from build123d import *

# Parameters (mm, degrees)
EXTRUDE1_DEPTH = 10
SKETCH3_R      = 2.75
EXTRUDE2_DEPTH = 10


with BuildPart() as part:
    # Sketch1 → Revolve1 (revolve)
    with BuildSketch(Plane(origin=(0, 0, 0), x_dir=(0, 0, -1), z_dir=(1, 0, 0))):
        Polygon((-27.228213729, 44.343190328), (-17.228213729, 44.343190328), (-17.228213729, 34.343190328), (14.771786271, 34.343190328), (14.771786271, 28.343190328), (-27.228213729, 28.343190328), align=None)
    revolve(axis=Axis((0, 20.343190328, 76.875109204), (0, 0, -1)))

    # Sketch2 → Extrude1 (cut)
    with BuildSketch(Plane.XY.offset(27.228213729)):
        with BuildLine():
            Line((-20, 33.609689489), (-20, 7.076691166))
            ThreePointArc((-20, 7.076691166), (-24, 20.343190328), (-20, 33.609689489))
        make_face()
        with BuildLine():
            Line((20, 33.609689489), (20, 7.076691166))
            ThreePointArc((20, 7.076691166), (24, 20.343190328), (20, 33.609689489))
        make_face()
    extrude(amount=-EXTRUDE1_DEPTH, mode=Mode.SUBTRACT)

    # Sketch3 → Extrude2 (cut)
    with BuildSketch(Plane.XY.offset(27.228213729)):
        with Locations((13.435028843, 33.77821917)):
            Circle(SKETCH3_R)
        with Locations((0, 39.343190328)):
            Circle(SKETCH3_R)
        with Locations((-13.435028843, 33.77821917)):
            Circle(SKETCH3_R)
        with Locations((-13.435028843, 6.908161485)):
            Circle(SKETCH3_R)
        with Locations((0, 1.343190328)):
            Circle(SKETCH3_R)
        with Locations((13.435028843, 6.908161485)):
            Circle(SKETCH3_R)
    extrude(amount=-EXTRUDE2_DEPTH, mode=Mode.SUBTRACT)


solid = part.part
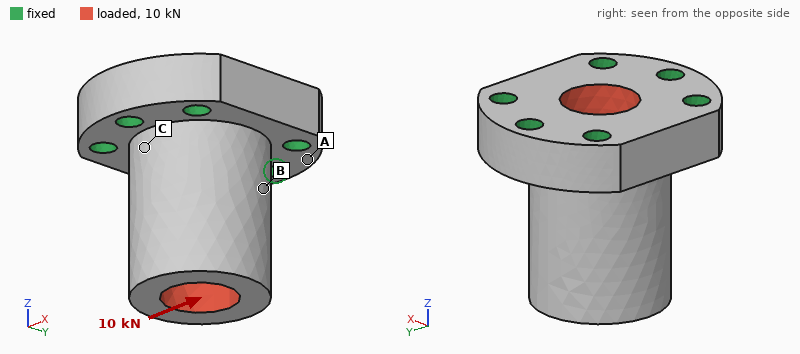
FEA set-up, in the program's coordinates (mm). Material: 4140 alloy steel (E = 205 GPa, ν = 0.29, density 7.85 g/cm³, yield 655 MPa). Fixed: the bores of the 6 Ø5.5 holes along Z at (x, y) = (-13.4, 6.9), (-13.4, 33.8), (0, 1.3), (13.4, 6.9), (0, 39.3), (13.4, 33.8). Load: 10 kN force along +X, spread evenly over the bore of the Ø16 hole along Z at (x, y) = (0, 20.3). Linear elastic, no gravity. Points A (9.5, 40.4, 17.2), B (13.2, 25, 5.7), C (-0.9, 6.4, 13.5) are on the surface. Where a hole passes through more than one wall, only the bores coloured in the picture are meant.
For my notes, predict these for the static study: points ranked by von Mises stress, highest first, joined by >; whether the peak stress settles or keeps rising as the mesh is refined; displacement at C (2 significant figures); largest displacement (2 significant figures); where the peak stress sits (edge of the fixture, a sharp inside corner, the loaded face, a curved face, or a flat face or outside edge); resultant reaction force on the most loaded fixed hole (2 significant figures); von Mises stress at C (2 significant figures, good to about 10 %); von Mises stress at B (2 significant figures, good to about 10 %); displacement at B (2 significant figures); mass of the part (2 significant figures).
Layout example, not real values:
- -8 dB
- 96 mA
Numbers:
- C > B > A
- keeps rising
- 3.3 µm
- 21 µm
- edge of the fixture
- 3.7 kN
- 35 MPa
- 24 MPa
- 10 µm
- 210 g
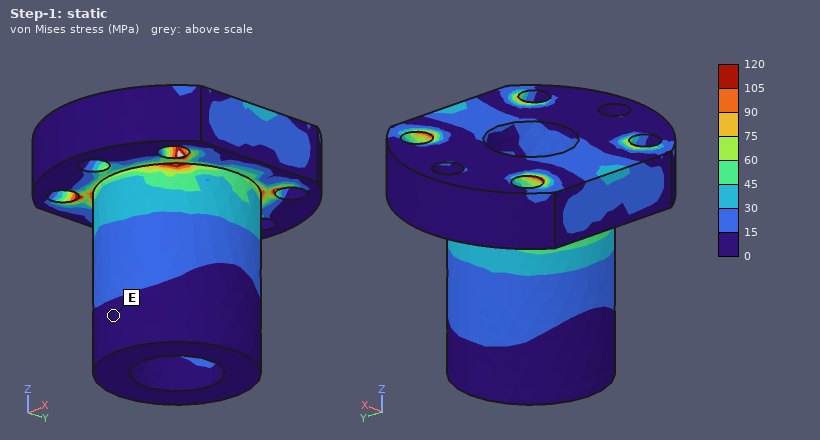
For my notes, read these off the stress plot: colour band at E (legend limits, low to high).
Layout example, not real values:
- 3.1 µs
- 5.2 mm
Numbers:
- 0 to 15 MPa
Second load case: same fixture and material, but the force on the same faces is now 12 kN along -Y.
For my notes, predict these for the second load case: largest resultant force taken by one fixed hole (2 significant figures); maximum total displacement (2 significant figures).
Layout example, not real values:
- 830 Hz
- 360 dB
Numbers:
- 3.7 kN
- 21 µm
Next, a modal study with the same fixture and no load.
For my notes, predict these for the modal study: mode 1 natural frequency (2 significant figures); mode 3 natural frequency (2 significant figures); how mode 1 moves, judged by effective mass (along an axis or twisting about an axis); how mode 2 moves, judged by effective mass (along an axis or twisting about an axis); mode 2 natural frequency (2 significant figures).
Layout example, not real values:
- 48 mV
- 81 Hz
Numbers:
- 11 kHz
- 23 kHz
- along X
- along Y
- 12 kHz
